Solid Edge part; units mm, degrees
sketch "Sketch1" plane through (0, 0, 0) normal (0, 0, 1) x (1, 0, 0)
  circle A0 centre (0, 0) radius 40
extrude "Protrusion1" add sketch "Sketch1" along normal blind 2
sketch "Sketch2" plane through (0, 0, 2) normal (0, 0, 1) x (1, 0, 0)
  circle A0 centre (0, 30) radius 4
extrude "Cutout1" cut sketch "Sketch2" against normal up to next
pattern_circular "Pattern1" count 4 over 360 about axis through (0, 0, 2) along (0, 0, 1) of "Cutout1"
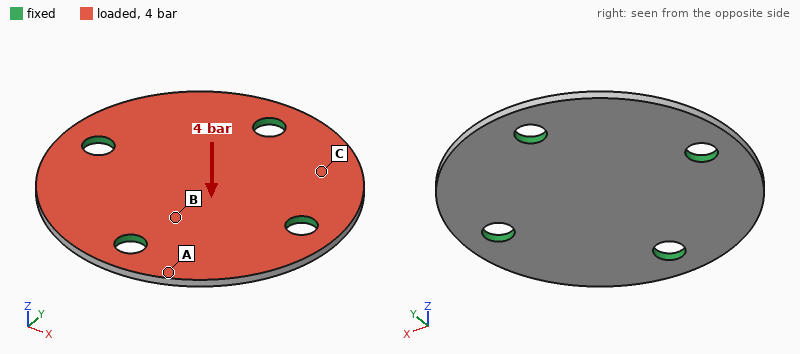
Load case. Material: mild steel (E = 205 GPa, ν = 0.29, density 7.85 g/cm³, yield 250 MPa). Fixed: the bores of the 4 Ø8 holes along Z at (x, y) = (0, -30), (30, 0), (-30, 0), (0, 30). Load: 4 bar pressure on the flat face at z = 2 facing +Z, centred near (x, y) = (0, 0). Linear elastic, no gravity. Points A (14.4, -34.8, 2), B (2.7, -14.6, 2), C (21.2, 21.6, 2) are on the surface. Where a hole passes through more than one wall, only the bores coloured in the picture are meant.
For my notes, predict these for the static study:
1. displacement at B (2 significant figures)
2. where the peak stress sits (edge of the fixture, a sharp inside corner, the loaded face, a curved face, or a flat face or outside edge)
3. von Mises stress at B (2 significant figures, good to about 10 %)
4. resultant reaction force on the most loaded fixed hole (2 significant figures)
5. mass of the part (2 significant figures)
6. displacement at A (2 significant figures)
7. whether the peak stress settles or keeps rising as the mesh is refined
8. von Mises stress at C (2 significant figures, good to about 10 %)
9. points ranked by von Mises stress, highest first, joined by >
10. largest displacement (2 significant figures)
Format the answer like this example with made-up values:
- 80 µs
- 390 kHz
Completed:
- 18 µm
- edge of the fixture
- 23 MPa
- 480 N
- 76 g
- 18 µm
- keeps rising
- 43 MPa
- C > B > A
- 42 µm
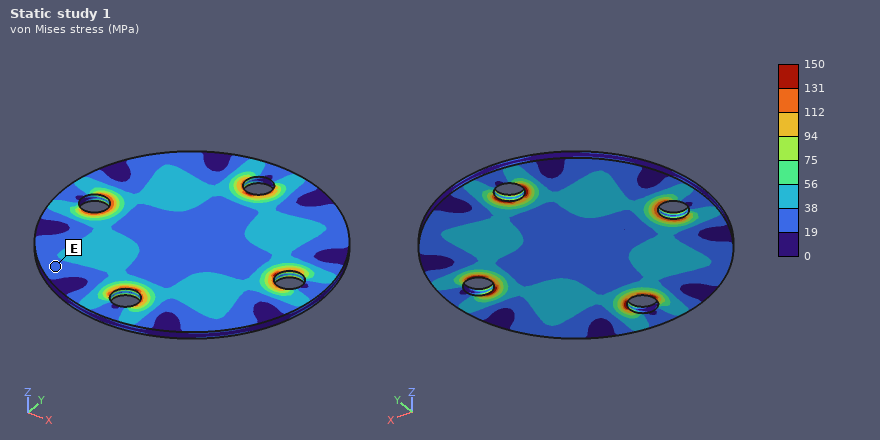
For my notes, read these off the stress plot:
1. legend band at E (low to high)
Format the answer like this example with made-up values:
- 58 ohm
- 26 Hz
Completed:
- 19 to 38 MPa
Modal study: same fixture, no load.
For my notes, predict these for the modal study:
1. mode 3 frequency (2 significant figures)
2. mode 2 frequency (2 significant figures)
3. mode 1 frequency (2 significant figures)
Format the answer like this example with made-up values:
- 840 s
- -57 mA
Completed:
- 5000 Hz
- 5000 Hz
- 5000 Hz
